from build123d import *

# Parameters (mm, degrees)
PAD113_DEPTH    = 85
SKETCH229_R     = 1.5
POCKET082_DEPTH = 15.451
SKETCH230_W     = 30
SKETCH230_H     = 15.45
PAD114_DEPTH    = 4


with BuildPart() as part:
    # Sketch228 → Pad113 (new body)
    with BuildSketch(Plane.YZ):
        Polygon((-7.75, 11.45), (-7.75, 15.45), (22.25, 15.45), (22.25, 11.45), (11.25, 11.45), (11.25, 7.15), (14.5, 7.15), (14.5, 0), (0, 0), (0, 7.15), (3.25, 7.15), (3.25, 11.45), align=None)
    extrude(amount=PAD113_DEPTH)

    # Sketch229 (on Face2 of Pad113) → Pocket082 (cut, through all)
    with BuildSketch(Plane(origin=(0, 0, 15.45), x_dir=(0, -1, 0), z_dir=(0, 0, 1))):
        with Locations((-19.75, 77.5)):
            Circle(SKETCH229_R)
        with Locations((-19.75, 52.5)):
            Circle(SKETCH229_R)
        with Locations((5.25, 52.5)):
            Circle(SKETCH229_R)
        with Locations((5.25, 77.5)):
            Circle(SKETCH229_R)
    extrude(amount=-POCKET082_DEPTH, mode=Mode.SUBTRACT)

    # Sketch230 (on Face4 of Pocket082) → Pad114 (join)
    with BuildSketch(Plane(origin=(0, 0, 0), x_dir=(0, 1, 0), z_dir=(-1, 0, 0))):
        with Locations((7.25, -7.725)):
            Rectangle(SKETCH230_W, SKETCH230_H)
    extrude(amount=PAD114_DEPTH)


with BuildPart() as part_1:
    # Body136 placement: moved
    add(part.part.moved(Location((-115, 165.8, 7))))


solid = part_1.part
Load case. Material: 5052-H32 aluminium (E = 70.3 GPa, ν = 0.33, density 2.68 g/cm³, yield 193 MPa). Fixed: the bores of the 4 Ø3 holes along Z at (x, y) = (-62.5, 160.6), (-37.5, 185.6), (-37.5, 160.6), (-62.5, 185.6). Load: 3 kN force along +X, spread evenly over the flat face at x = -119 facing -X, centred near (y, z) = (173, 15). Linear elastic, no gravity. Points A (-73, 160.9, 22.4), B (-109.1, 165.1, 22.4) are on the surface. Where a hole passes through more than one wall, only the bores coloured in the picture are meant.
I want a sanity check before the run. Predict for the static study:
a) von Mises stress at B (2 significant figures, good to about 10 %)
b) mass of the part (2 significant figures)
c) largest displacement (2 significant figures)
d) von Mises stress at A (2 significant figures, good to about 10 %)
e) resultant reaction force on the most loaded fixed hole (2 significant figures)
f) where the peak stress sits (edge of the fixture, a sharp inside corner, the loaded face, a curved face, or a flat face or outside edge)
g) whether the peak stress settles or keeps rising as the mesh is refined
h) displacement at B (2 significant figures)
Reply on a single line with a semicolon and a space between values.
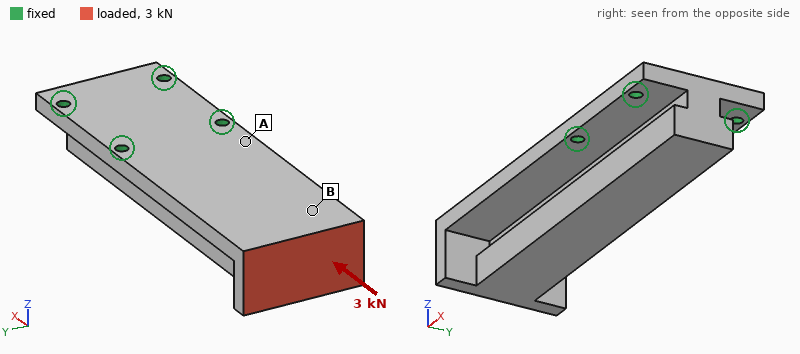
5.3 MPa; 63 g; 87 µm; 13 MPa; 1.1 kN; edge of the fixture; keeps rising; 58 µm
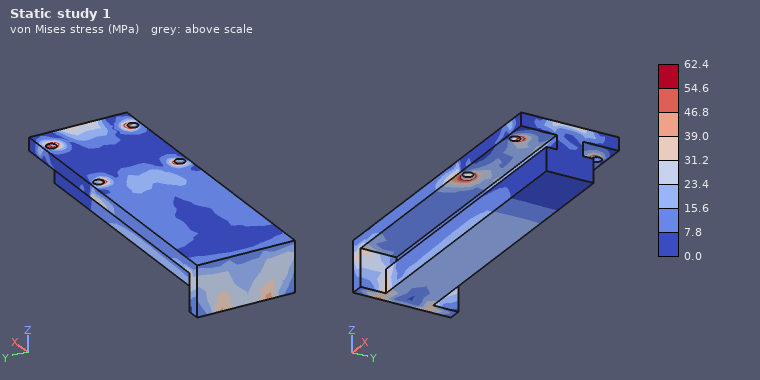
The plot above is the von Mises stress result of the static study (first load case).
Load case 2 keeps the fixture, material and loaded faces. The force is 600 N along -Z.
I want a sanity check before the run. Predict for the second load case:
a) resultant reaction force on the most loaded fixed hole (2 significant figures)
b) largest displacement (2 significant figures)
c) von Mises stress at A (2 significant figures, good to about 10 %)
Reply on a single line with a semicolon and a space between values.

1.1 kN; 0.23 mm; 36 MPa
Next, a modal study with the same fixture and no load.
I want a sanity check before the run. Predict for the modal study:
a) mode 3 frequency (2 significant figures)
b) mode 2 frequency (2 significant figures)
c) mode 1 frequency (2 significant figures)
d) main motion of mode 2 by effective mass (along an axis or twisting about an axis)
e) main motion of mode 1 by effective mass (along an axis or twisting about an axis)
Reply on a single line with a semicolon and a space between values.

6100 Hz; 4000 Hz; 2100 Hz; along Y; along Z
